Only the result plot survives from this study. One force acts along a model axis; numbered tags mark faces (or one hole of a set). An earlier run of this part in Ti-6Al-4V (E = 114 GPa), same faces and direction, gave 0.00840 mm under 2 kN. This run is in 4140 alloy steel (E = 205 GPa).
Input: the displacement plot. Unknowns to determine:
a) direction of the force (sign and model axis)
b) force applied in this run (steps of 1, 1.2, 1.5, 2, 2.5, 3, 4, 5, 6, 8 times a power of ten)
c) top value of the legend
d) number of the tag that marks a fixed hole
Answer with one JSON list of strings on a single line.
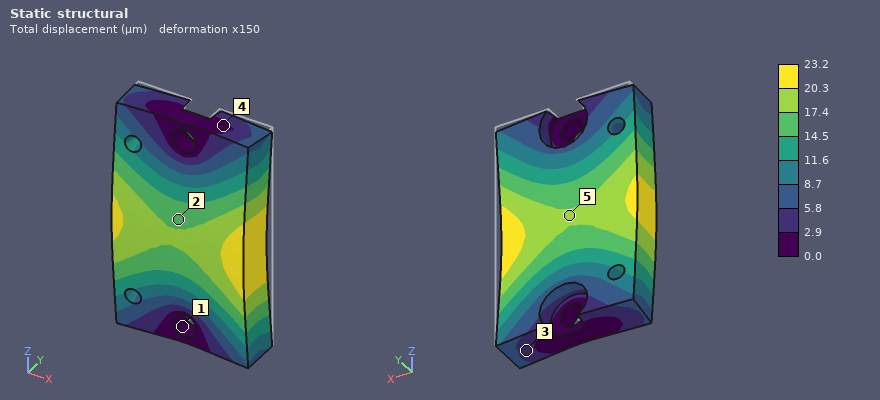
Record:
["-Y", "10 kN", "23.2 µm", "1"]
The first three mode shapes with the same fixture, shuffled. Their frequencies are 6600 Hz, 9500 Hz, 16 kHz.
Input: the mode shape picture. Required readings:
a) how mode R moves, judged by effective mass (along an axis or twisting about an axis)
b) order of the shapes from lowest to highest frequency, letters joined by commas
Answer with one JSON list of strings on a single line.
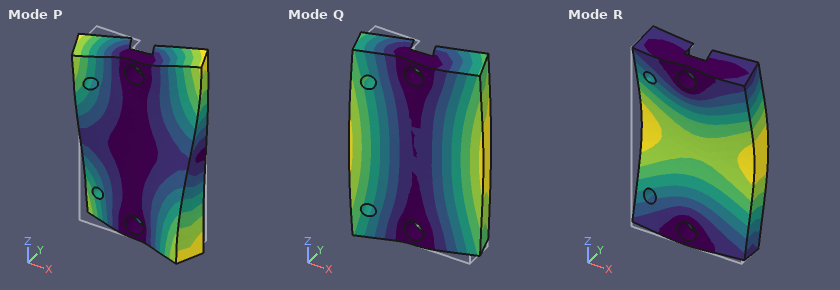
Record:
["along Y", "Q, R, P"]
